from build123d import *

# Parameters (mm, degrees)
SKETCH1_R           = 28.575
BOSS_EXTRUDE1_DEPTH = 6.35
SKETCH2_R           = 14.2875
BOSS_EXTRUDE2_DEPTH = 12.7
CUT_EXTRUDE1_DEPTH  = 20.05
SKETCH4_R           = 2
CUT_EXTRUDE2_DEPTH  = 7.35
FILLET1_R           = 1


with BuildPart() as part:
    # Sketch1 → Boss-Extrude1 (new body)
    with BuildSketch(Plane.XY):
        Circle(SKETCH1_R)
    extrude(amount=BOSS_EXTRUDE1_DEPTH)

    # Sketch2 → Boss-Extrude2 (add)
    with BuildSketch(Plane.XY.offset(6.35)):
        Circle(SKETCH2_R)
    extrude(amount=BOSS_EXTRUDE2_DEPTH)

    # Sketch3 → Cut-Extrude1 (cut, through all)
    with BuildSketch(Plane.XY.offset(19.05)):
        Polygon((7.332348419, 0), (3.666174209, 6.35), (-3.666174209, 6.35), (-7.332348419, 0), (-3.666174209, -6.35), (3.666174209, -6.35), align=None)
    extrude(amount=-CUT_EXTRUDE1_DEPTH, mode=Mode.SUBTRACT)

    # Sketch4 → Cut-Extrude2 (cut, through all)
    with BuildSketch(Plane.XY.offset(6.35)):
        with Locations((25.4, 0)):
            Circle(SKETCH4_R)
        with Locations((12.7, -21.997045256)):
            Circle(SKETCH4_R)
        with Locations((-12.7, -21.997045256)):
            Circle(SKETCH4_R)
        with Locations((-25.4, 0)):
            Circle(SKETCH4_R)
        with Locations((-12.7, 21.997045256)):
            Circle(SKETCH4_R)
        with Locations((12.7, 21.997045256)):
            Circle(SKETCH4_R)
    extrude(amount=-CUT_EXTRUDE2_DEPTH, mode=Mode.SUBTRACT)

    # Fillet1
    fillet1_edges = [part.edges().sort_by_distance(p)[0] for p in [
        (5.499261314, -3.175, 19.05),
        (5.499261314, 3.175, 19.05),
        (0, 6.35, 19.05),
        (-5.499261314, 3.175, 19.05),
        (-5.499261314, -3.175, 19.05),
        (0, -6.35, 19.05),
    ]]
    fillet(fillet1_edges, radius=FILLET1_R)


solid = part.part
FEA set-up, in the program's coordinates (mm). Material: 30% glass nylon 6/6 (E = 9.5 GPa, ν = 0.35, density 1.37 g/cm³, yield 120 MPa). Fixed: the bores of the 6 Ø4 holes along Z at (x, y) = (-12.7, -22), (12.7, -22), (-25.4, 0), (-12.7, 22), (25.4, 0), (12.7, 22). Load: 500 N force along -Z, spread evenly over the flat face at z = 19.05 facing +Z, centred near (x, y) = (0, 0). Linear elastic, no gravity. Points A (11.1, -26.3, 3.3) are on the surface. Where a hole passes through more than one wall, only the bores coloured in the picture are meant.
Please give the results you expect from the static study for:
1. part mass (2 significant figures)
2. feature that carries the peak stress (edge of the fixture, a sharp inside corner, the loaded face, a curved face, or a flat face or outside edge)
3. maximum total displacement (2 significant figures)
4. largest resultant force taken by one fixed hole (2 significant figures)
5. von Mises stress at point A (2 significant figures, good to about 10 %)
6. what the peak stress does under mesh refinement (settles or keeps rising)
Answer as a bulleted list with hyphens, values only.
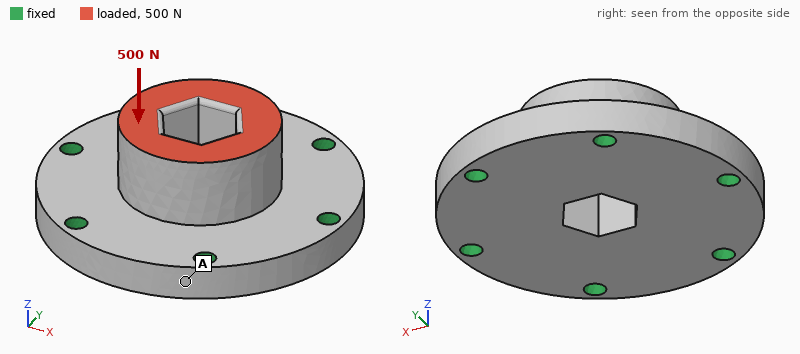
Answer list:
- 29 g
- edge of the fixture
- 11 µm
- 90 N
- 1.4 MPa
- keeps rising
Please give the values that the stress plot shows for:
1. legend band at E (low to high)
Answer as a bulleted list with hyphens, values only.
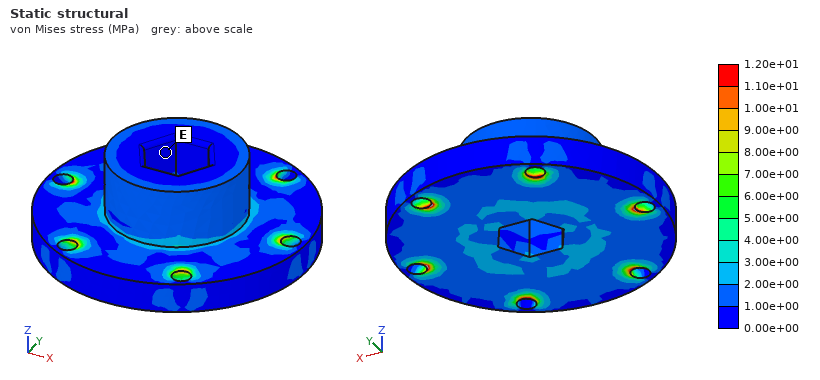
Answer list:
- 0.00e+00 to 1.00e+00 MPa
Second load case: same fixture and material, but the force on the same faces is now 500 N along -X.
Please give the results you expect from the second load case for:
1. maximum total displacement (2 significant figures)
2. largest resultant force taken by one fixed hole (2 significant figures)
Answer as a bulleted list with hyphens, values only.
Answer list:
- 23 µm
- 170 N
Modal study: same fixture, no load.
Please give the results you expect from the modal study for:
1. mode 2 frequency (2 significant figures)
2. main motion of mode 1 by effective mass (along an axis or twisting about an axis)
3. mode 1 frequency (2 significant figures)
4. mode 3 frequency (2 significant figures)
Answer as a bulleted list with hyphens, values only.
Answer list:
- 11 kHz
- along Z
- 8900 Hz
- 11 kHz
